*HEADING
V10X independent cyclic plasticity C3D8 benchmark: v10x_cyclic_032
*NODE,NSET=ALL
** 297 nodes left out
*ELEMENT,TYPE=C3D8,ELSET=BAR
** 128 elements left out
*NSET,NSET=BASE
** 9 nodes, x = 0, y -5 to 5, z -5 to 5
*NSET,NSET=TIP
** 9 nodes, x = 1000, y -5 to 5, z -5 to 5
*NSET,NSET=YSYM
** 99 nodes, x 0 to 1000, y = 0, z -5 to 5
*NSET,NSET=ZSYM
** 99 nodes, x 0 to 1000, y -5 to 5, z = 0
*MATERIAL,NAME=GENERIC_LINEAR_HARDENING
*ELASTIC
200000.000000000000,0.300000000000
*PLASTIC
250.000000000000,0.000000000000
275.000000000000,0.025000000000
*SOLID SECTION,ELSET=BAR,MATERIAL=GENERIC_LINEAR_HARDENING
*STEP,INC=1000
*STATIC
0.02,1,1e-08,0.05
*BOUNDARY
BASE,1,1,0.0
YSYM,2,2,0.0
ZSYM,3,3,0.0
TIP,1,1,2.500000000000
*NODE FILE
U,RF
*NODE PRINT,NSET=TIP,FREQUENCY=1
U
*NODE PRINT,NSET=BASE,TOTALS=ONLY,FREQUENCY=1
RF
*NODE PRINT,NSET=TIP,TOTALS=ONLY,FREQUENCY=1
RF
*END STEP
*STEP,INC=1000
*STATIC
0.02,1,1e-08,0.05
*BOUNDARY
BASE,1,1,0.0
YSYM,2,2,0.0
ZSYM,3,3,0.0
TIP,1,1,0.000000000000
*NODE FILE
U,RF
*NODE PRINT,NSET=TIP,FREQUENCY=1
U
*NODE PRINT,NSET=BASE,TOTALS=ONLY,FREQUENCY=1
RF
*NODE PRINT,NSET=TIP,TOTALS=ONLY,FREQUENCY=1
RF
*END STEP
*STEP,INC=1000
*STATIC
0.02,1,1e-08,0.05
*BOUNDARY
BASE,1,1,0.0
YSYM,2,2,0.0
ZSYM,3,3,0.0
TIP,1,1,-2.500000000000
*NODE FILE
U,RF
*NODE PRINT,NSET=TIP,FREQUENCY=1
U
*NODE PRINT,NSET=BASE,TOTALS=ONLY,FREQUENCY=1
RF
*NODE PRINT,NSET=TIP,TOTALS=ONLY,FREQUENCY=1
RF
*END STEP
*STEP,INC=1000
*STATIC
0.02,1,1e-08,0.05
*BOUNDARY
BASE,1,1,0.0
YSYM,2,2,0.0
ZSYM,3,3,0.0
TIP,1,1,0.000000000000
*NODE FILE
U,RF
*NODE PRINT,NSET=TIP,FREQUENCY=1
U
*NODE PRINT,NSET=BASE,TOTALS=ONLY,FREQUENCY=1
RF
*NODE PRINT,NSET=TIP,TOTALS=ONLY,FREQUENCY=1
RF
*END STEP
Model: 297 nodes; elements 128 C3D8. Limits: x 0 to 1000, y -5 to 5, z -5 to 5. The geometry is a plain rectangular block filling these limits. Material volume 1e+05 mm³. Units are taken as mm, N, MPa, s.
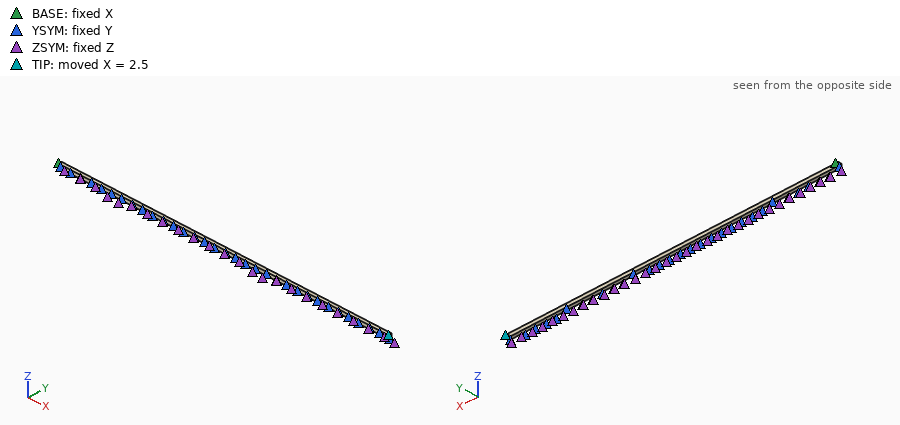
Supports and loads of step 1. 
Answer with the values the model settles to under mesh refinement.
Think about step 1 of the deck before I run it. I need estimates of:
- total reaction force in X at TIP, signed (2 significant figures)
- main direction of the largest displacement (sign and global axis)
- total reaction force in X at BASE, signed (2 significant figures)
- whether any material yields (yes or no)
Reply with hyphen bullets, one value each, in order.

- 25000 N
- +X
- -25000 N
- yes
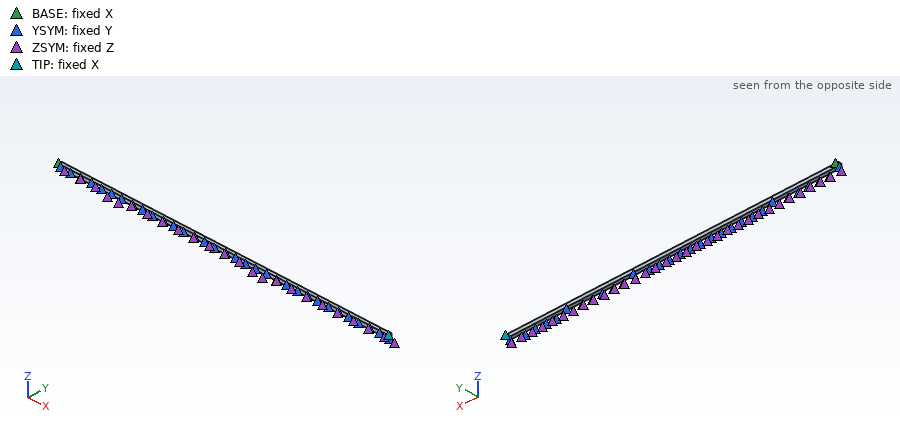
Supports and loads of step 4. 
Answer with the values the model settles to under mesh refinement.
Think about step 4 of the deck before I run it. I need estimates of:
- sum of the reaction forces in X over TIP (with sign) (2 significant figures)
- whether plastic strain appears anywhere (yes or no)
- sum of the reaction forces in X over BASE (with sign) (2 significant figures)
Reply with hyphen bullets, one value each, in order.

- 25000 N
- yes
- -25000 N
